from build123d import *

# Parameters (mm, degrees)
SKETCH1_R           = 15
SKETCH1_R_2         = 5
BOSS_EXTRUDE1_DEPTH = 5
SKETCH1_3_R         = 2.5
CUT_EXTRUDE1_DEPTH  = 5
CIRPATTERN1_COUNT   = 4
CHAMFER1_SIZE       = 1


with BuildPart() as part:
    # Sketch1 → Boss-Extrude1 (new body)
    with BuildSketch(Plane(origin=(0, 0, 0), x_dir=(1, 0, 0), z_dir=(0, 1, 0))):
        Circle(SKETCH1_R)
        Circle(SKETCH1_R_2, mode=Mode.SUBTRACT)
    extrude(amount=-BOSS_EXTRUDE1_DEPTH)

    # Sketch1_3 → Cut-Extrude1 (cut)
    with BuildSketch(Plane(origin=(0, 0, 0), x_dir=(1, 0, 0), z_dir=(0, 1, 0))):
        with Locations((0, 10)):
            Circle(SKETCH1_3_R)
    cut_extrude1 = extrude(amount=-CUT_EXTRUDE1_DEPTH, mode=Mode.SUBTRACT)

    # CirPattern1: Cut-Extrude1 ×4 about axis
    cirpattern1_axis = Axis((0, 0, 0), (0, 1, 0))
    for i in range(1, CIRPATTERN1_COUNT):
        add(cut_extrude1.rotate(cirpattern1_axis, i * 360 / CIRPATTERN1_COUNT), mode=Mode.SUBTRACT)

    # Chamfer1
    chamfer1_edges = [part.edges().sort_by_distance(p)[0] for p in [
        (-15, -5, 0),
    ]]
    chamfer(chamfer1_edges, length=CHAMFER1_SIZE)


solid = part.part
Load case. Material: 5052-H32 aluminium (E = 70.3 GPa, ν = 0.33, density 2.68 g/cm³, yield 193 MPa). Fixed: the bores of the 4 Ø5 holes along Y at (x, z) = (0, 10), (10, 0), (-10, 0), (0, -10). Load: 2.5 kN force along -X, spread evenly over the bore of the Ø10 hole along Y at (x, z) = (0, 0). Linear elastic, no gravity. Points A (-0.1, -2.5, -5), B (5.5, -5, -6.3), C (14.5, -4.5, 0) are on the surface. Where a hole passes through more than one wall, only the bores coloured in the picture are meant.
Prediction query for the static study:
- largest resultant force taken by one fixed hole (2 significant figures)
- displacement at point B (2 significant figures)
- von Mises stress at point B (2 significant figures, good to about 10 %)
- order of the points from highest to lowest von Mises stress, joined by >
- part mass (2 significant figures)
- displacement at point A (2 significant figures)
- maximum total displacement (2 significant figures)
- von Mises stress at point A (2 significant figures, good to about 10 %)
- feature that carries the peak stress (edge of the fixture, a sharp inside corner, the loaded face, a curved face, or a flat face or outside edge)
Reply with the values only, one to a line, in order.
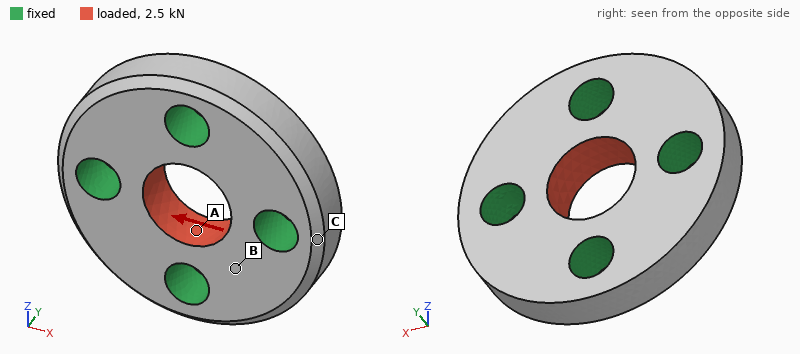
740 N
0.80 µm
7.6 MPa
A > B > C
7.2 g
1.5 µm
1.5 µm
28 MPa
edge of the fixture
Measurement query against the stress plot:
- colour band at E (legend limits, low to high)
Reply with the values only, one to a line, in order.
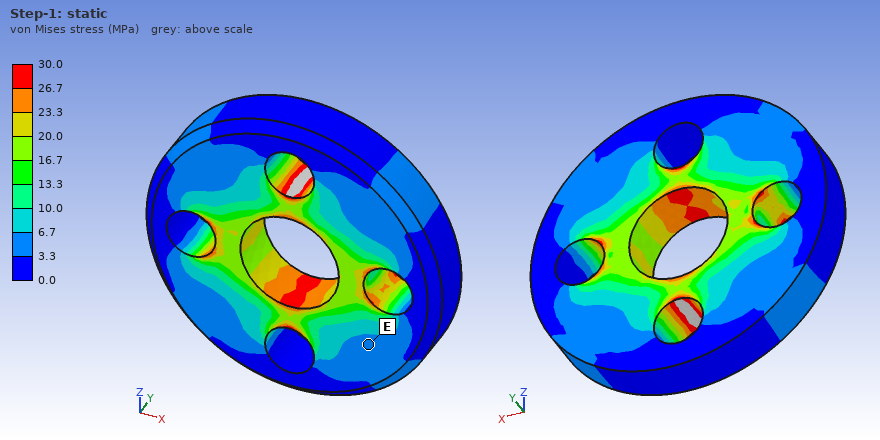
3.3 to 6.7 MPa
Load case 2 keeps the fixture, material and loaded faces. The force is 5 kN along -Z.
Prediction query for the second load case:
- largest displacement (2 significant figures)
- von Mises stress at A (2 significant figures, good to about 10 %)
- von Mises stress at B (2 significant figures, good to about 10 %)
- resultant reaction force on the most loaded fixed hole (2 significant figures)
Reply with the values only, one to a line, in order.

3.0 µm
43 MPa
16 MPa
1.5 kN
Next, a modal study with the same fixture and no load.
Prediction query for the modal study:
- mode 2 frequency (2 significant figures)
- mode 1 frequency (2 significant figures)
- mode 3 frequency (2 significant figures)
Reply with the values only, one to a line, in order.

73 kHz
72 kHz
73 kHz
